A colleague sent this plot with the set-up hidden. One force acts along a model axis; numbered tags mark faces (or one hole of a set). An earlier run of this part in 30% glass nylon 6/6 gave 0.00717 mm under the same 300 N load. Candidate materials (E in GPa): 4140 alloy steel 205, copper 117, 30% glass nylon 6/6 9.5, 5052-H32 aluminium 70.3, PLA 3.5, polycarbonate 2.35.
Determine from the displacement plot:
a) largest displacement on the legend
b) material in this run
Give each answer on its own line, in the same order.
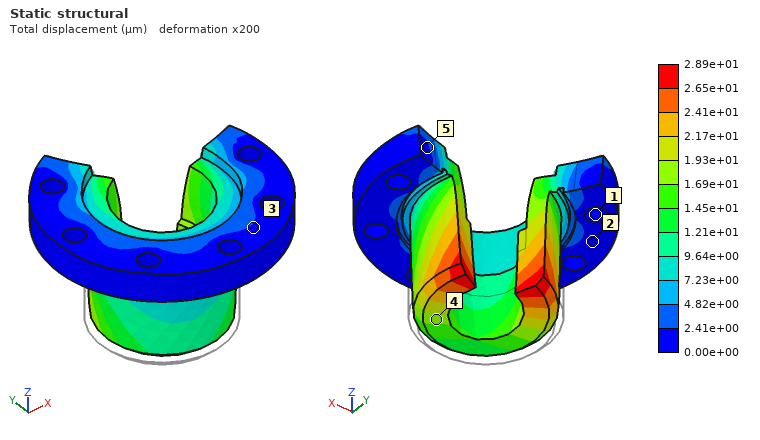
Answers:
2.89e+01 µm
polycarbonate
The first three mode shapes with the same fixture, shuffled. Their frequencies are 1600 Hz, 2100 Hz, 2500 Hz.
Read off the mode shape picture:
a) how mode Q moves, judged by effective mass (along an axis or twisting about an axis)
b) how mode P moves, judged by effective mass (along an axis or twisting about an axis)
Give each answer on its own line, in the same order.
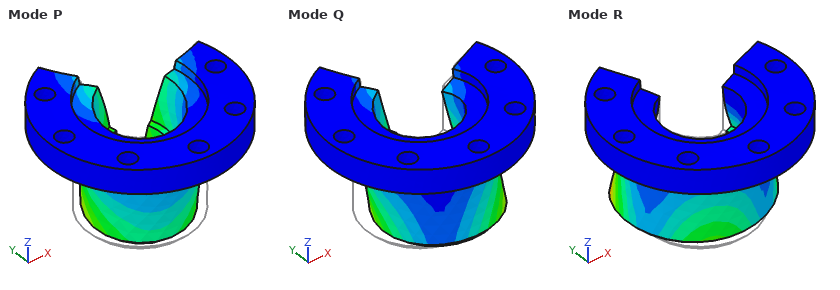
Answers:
along X
along Y
